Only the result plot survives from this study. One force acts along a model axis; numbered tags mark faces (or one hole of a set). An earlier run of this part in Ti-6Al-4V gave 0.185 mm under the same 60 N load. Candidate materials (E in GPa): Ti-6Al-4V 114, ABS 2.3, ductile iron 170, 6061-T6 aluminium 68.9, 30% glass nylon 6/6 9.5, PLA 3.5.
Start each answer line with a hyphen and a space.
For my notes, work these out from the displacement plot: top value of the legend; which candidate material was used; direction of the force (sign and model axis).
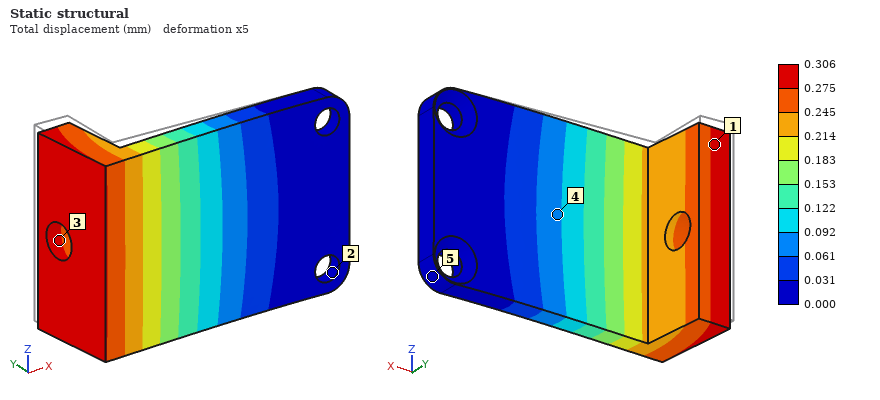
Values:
- 0.306 mm
- 6061-T6 aluminium
- -Y
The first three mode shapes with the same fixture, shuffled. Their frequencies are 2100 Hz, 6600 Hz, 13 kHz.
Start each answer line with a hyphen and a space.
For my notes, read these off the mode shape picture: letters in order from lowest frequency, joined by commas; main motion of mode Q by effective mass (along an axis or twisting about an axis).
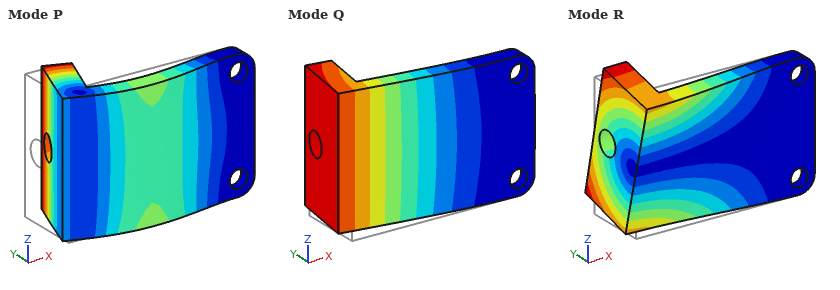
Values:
- Q, R, P
- along Y
